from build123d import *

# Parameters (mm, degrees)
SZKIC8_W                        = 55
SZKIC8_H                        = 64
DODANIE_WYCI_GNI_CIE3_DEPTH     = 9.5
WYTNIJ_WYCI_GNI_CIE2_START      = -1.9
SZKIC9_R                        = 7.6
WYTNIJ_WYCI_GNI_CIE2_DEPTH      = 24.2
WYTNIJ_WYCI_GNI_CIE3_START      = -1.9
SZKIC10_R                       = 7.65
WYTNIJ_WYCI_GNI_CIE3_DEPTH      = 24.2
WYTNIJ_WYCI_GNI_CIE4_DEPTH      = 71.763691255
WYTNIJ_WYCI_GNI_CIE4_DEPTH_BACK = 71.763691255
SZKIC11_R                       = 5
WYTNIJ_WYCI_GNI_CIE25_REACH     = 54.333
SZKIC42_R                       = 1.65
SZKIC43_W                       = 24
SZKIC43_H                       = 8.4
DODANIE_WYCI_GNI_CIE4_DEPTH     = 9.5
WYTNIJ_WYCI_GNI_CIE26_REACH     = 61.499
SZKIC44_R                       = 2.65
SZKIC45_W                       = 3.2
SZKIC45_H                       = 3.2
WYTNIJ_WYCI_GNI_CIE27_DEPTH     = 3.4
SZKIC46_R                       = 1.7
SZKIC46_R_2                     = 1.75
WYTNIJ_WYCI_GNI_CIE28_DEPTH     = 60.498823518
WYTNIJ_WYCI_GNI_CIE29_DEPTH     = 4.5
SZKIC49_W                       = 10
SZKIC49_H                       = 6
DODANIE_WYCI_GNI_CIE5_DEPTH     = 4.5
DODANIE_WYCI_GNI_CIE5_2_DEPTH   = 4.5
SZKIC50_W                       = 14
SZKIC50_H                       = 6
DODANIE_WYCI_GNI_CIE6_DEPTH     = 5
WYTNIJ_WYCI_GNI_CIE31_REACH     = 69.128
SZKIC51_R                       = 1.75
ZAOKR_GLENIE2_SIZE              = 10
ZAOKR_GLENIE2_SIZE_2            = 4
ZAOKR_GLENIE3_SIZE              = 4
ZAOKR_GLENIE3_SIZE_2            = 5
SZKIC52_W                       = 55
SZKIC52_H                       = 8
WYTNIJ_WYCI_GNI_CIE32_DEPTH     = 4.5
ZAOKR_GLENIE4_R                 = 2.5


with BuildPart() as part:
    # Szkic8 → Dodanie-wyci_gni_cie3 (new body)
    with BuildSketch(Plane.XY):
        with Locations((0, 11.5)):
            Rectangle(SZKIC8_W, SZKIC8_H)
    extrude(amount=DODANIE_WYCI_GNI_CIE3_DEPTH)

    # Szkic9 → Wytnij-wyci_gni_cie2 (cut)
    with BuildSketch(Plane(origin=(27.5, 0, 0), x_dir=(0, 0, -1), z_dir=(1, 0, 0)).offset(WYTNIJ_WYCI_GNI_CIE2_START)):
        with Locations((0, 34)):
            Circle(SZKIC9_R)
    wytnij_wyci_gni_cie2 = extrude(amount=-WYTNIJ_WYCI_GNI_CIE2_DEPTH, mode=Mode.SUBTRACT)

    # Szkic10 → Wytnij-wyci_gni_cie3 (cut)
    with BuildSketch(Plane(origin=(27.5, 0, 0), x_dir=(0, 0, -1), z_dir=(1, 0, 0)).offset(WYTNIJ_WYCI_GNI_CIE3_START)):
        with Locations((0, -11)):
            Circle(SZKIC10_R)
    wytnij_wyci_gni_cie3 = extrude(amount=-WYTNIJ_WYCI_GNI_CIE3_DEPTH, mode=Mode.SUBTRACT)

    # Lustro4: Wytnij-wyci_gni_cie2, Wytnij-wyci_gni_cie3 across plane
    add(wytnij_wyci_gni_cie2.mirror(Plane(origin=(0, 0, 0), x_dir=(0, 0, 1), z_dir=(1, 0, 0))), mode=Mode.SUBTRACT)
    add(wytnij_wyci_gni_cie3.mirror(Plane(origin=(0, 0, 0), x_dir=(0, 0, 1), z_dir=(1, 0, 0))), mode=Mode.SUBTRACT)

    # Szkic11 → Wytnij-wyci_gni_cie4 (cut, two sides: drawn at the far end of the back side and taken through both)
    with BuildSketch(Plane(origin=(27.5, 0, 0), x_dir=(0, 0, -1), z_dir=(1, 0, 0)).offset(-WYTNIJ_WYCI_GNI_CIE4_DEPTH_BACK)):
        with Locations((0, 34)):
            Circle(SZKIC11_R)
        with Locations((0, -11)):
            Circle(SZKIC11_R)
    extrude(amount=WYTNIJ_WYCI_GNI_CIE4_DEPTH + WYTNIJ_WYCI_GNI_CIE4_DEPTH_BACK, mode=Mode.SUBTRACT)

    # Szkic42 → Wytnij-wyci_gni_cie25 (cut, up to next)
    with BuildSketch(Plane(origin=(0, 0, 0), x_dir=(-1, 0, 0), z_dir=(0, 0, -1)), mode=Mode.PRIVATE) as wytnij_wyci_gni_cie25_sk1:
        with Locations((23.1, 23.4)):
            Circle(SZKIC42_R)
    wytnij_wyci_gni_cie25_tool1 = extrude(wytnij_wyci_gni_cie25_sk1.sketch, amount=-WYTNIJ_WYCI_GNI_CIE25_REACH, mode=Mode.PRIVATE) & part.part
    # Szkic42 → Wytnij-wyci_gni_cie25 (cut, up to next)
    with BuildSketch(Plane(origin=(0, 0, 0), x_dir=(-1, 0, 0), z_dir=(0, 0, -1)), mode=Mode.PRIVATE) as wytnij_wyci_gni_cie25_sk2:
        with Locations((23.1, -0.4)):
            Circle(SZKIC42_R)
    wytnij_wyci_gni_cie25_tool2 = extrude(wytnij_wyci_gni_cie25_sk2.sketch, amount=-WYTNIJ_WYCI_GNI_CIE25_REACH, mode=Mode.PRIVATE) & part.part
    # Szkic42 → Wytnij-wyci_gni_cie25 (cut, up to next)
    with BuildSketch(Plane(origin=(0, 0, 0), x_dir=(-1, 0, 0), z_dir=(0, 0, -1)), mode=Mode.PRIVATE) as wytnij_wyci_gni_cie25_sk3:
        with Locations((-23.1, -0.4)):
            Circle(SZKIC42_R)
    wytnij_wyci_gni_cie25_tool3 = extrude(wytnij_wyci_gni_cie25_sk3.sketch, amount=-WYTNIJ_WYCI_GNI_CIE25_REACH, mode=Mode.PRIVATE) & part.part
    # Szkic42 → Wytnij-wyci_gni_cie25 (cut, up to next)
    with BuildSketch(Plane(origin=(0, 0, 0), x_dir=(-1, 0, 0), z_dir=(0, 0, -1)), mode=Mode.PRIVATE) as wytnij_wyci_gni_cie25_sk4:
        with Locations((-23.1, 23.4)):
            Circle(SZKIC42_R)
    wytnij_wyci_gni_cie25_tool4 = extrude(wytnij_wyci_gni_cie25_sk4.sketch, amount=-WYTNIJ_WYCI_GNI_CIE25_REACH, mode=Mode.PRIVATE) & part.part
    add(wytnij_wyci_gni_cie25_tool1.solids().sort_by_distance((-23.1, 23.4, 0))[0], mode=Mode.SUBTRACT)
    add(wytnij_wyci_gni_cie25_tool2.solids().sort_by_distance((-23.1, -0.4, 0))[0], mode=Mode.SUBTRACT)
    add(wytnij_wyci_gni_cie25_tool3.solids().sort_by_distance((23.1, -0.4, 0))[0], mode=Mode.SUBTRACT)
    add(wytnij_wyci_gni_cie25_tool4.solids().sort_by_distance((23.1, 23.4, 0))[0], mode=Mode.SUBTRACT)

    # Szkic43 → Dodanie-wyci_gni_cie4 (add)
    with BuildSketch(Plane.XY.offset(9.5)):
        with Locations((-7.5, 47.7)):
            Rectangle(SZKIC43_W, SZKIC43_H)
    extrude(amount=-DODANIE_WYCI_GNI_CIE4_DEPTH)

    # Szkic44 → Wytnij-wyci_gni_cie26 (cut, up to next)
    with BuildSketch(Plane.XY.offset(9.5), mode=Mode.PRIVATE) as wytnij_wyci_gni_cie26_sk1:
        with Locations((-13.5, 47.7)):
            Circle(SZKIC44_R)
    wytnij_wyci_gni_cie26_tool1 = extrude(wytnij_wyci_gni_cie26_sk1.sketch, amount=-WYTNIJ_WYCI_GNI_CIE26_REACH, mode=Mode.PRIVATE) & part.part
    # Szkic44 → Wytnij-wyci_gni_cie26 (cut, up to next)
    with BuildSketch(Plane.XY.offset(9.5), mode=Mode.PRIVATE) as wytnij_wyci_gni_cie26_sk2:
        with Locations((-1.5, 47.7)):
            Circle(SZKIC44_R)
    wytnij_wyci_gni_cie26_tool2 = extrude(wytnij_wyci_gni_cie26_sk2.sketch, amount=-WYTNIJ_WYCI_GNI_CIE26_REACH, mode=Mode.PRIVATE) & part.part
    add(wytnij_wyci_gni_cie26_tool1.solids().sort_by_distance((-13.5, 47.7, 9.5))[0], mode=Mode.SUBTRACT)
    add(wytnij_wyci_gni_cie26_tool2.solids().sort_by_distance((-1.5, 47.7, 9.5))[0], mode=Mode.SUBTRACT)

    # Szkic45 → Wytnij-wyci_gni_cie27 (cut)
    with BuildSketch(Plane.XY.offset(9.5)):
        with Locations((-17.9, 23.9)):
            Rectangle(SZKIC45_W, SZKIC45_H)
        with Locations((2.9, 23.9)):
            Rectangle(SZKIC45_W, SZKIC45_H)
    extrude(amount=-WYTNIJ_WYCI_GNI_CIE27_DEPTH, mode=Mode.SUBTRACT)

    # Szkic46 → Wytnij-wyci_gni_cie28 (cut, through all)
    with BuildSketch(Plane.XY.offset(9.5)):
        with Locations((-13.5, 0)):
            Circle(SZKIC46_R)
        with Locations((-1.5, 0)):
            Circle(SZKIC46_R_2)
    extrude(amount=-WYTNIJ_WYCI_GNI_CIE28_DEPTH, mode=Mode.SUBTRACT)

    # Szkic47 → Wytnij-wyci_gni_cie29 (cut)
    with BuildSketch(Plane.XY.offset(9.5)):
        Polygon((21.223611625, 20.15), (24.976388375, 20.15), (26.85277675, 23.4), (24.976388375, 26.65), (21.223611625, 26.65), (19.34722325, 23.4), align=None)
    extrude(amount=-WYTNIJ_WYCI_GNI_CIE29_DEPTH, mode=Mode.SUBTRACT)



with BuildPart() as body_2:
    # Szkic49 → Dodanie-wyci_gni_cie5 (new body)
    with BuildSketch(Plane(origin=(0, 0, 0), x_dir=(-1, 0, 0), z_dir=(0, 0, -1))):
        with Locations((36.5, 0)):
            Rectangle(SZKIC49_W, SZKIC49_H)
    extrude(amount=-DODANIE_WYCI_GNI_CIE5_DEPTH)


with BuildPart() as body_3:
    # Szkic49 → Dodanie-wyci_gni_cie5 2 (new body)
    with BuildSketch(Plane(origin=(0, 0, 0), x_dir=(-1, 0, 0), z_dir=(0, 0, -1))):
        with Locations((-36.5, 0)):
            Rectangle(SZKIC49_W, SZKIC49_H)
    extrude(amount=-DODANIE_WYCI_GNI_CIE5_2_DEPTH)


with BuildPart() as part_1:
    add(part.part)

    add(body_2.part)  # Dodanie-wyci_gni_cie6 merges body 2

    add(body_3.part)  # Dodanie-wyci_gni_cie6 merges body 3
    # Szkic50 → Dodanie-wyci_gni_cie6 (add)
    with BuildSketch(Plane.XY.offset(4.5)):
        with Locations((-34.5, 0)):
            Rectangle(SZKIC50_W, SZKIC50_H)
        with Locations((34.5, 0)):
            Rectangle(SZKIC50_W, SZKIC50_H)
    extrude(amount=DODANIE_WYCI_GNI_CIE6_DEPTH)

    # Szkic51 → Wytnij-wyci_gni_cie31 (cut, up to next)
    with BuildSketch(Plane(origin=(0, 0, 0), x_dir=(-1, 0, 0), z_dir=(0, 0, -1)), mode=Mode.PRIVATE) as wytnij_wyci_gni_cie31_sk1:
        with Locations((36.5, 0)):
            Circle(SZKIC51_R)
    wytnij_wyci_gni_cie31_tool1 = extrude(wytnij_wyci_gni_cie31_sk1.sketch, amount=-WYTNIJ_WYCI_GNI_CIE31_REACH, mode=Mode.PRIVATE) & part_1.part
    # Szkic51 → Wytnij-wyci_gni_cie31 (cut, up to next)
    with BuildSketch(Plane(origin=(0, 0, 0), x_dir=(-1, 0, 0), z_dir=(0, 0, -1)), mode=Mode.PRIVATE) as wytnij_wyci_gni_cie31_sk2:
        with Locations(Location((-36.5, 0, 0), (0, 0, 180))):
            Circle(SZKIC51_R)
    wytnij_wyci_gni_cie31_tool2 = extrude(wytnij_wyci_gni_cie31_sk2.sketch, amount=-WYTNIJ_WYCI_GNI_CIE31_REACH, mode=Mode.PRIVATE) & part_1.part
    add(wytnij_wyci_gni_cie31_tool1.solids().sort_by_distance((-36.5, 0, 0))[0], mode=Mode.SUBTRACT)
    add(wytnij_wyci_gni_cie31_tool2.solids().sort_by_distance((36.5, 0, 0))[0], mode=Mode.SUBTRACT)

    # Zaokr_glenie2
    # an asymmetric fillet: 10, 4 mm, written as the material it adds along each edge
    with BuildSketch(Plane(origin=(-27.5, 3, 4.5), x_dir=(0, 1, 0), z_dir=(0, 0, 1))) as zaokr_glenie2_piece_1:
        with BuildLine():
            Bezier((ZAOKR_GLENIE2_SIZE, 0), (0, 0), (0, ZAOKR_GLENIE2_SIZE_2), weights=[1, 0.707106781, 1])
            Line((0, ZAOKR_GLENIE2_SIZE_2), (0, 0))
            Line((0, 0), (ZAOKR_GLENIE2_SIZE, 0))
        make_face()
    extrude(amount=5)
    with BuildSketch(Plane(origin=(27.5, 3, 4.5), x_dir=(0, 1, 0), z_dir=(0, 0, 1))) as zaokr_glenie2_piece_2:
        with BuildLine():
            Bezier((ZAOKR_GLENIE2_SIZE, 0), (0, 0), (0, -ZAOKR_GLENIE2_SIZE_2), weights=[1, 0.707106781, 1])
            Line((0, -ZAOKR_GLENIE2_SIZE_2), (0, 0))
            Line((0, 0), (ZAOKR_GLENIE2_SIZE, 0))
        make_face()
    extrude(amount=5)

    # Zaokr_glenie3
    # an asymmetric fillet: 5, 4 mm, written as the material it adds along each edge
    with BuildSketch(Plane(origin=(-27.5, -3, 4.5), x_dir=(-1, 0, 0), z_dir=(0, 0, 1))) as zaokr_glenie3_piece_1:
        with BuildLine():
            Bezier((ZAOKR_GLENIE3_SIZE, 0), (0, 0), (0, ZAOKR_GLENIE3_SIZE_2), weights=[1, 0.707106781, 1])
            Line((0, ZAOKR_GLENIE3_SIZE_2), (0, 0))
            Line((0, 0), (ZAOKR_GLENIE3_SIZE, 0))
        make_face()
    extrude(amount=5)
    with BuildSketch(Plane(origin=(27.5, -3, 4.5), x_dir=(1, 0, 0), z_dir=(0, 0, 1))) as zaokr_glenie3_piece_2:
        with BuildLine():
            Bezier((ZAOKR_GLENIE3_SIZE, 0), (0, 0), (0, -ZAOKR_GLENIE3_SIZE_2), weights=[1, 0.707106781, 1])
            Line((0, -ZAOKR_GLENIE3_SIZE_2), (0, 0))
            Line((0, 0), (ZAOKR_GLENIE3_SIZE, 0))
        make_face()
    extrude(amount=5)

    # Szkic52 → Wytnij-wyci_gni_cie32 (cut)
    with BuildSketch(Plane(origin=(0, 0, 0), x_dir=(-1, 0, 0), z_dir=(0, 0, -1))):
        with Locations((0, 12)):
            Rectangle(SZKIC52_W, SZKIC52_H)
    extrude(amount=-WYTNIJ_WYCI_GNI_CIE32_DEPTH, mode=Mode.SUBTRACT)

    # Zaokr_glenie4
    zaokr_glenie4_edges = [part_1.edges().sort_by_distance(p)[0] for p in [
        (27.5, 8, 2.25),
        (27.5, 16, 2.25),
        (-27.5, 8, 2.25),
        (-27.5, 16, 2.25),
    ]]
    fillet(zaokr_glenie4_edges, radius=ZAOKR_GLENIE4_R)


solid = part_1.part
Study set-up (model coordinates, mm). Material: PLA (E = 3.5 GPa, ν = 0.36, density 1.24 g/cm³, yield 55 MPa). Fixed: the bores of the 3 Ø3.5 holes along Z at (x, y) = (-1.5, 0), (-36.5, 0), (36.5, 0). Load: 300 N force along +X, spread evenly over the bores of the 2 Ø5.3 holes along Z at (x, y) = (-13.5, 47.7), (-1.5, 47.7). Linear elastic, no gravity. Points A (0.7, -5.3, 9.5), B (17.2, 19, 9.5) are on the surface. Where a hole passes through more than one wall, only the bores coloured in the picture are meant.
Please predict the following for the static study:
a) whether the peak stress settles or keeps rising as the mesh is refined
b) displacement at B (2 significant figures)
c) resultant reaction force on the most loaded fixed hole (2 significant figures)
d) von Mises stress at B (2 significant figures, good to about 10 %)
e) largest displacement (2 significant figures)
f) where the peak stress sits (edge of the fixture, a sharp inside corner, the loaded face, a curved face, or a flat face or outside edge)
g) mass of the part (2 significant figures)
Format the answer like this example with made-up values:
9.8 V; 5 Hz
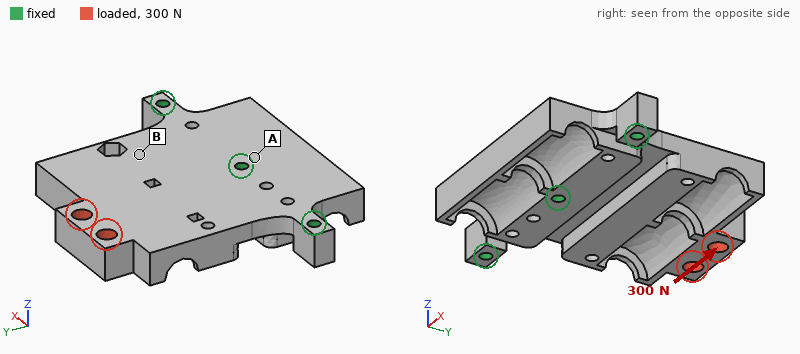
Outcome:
keeps rising; 0.079 mm; 230 N; 3.4 MPa; 0.31 mm; edge of the fixture; 30 g
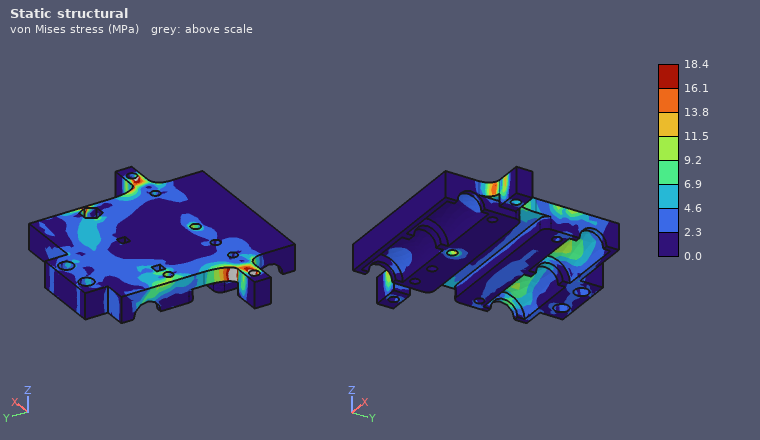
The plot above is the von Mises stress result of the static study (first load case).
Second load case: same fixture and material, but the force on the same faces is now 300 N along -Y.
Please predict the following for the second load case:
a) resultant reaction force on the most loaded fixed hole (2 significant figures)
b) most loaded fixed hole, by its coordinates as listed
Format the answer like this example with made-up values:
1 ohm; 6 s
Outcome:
250 N; (-1.5, 0)
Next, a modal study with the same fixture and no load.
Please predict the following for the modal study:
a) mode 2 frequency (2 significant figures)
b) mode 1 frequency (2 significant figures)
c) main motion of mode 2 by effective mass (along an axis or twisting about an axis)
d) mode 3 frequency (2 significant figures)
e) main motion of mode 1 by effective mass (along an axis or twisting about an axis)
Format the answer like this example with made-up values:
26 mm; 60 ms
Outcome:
1500 Hz; 610 Hz; twisting about Y; 2000 Hz; along Z
